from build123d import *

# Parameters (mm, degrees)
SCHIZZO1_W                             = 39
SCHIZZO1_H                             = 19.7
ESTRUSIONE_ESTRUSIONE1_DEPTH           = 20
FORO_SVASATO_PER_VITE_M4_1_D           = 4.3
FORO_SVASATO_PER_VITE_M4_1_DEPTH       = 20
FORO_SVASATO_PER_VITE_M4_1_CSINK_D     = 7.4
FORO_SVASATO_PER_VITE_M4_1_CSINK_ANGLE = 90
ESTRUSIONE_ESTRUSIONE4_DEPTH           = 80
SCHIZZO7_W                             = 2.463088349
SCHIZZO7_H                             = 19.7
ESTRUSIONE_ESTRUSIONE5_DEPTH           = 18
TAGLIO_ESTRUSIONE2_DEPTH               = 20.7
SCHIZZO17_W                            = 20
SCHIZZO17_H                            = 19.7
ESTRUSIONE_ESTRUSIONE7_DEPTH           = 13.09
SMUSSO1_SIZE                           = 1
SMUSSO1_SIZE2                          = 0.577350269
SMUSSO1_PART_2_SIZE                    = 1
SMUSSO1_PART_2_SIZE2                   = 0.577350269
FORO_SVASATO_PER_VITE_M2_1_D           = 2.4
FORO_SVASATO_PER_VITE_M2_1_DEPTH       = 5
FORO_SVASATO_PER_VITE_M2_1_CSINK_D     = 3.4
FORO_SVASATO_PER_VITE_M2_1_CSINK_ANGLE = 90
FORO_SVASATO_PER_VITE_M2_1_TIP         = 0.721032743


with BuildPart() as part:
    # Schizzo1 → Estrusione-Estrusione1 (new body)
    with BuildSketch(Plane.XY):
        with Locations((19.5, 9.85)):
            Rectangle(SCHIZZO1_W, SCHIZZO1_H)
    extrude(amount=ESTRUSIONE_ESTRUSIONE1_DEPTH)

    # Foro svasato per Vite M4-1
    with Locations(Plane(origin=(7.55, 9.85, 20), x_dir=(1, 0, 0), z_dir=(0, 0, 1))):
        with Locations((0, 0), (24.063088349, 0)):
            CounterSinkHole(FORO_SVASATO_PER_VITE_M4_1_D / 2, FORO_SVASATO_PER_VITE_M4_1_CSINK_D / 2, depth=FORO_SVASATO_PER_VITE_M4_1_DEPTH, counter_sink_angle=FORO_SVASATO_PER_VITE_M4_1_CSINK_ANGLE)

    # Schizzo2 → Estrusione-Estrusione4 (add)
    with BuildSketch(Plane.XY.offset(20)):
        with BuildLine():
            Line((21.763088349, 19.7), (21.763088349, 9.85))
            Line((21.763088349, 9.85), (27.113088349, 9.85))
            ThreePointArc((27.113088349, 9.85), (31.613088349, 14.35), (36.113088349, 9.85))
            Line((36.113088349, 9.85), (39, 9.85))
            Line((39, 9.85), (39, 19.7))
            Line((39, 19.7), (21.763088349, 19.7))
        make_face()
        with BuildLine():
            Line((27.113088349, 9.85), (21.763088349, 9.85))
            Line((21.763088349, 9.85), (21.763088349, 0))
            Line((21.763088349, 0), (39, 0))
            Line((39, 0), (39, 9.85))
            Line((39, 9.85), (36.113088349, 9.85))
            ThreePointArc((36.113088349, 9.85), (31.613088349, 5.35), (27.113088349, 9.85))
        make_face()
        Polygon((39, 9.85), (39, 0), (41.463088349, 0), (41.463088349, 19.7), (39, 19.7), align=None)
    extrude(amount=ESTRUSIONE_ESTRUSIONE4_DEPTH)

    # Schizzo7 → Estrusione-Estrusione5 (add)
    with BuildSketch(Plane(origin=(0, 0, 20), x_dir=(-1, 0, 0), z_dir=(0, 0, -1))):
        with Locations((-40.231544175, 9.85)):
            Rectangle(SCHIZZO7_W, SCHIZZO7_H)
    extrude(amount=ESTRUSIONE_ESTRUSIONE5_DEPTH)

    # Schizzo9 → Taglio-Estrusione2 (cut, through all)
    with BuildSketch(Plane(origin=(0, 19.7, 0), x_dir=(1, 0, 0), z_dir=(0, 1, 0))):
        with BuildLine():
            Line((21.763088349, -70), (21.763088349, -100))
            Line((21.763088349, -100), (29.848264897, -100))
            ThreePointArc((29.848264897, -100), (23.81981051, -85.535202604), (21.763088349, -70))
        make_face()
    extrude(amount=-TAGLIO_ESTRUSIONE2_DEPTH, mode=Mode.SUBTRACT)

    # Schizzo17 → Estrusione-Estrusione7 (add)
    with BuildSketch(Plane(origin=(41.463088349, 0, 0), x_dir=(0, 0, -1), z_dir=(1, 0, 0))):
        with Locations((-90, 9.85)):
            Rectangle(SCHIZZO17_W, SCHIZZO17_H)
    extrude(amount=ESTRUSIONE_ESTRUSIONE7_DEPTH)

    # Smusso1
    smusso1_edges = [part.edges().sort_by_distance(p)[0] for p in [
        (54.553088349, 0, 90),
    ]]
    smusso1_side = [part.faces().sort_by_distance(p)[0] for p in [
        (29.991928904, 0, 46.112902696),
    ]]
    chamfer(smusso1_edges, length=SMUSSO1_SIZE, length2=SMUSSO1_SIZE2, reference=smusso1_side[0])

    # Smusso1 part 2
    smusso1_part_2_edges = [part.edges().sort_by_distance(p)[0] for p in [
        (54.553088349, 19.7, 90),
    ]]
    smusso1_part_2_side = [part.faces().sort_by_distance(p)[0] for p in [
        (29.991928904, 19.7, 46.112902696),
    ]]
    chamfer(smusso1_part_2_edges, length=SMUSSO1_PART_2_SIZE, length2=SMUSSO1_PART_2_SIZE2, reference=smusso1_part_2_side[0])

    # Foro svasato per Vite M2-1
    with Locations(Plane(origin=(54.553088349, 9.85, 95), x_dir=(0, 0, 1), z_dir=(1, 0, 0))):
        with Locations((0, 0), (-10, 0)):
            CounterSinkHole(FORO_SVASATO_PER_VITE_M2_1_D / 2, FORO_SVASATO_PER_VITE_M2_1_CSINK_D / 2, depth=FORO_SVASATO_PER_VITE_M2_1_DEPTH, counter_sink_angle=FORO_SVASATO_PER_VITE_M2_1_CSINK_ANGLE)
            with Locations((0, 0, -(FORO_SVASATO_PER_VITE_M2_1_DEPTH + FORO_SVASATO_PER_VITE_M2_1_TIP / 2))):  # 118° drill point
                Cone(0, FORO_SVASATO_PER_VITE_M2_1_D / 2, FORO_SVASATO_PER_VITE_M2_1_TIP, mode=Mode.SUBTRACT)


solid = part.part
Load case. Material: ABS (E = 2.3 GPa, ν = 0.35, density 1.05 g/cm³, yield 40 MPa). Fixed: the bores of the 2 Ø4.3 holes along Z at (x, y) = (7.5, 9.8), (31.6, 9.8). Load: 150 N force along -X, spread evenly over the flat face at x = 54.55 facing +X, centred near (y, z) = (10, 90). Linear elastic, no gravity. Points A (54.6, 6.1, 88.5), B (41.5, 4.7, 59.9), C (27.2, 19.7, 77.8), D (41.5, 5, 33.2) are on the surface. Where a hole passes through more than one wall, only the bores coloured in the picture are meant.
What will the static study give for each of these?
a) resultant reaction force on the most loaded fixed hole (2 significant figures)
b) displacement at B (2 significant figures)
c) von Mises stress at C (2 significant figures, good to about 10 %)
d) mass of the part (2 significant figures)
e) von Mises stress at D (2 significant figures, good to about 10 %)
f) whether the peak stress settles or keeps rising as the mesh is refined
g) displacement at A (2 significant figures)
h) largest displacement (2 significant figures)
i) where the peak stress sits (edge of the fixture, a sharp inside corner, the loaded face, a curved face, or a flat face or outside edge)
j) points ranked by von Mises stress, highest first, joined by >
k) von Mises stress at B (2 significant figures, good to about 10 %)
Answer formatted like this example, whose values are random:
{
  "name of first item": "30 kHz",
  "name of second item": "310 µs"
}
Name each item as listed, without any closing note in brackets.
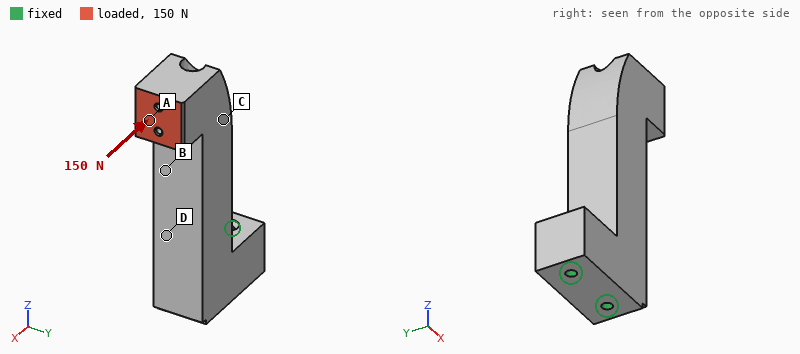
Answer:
{
  "resultant reaction force on the most loaded fixed hole": "330 N",
  "displacement at B": "0.48 mm",
  "von Mises stress at C": "1.5 MPa",
  "mass of the part": "47 g",
  "von Mises stress at D": "7.0 MPa",
  "whether the peak stress settles or keeps rising as the mesh is refined": "keeps rising",
  "displacement at A": "1.0 mm",
  "largest displacement": "1.2 mm",
  "where the peak stress sits": "edge of the fixture",
  "points ranked by von Mises stress, highest first, joined by >": "D > B > C > A",
  "von Mises stress at B": "3.7 MPa"
}
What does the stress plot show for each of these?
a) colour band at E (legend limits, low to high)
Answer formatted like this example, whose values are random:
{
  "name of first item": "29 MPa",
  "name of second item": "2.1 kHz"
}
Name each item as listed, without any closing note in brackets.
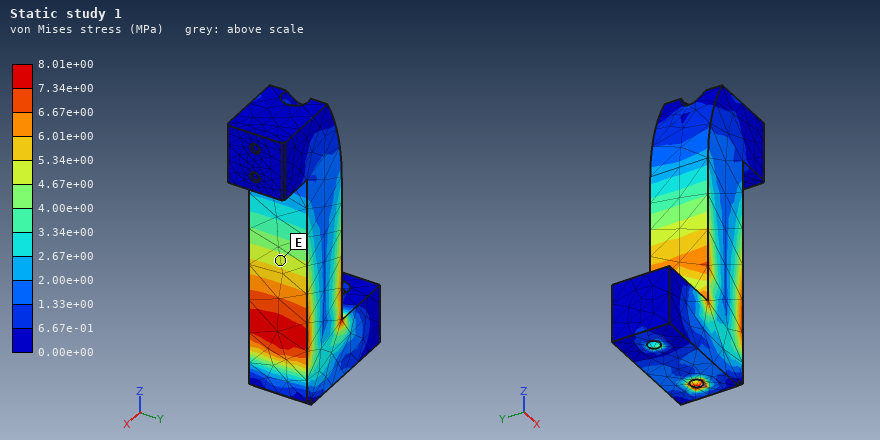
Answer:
{
  "colour band at E": "4.67e+00 to 5.34e+00 MPa"
}
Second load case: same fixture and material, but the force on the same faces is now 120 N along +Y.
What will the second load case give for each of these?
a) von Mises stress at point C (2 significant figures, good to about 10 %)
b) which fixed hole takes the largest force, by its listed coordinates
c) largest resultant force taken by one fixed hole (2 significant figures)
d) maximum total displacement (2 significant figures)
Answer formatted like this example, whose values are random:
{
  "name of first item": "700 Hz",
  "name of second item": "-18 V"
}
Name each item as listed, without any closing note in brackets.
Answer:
{
  "von Mises stress at point C": "2.2 MPa",
  "which fixed hole takes the largest force, by its listed coordinates": "(31.6, 9.8)",
  "largest resultant force taken by one fixed hole": "210 N",
  "maximum total displacement": "1.3 mm"
}
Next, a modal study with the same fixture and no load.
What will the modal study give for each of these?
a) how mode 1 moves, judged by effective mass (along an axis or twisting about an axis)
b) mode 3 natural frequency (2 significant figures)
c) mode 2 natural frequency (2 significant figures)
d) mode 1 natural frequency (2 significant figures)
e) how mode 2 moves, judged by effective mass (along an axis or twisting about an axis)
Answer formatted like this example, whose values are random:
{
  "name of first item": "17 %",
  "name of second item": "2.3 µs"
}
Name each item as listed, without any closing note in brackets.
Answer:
{
  "how mode 1 moves, judged by effective mass": "along Y",
  "mode 3 natural frequency": "1800 Hz",
  "mode 2 natural frequency": "510 Hz",
  "mode 1 natural frequency": "480 Hz",
  "how mode 2 moves, judged by effective mass": "along X"
}
